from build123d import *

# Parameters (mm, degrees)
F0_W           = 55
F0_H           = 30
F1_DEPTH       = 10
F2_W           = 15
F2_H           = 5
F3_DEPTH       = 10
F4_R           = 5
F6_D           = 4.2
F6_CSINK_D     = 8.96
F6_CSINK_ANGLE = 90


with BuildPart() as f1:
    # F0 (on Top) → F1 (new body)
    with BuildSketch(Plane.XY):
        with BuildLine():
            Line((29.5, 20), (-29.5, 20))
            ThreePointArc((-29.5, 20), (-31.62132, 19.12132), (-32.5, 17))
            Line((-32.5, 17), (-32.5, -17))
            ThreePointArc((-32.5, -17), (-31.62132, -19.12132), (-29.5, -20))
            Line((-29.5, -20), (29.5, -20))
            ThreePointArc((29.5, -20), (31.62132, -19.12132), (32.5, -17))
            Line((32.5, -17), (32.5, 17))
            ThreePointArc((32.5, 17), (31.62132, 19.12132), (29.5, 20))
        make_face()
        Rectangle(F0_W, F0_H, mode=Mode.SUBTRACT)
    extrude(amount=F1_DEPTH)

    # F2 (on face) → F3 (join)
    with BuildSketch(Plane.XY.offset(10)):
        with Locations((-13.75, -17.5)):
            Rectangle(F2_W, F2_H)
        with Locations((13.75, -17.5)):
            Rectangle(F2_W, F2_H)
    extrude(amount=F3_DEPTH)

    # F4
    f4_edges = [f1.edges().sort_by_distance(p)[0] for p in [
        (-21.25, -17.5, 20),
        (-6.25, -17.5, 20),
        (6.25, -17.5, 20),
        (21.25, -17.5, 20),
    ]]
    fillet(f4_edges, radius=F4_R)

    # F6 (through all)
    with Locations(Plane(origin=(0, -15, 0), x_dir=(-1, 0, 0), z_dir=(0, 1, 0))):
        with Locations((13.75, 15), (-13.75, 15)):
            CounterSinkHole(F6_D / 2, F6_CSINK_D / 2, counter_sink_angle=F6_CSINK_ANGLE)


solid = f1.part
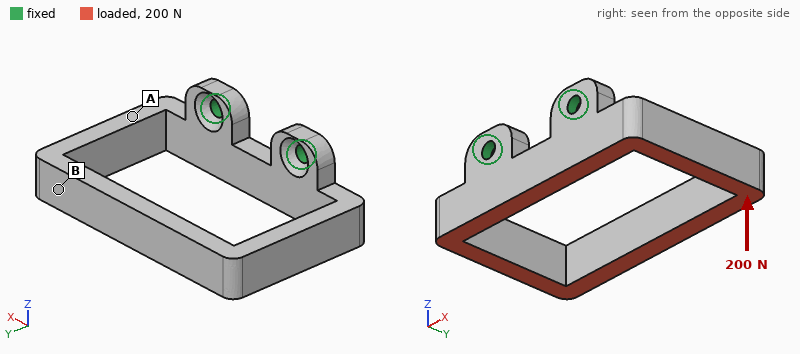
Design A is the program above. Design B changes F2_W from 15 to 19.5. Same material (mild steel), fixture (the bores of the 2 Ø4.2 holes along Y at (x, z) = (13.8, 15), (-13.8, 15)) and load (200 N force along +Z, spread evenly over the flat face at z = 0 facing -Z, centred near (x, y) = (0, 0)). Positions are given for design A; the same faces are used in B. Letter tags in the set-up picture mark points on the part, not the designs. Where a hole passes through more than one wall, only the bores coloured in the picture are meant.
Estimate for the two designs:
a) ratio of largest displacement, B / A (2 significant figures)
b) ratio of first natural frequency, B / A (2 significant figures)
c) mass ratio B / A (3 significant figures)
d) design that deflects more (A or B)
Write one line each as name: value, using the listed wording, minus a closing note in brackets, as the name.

ratio of largest displacement, B / A: 0.89
ratio of first natural frequency, B / A: 1.1
mass ratio B / A: 1.04
design that deflects more: A
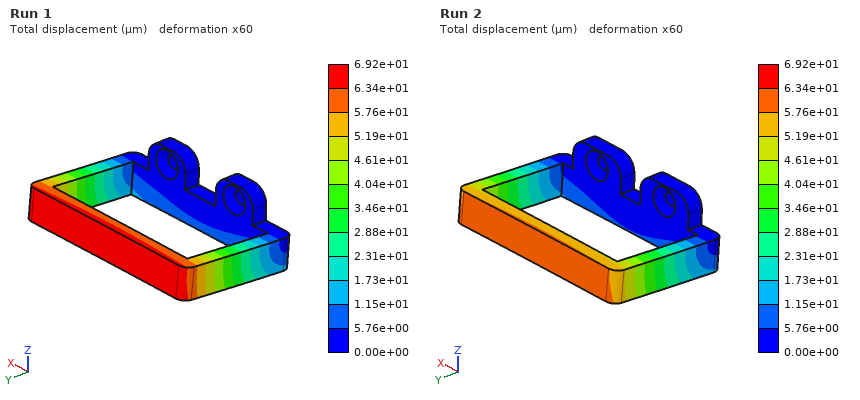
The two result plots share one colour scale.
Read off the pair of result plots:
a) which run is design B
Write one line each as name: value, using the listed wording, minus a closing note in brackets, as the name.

which run is design B: Run 2
